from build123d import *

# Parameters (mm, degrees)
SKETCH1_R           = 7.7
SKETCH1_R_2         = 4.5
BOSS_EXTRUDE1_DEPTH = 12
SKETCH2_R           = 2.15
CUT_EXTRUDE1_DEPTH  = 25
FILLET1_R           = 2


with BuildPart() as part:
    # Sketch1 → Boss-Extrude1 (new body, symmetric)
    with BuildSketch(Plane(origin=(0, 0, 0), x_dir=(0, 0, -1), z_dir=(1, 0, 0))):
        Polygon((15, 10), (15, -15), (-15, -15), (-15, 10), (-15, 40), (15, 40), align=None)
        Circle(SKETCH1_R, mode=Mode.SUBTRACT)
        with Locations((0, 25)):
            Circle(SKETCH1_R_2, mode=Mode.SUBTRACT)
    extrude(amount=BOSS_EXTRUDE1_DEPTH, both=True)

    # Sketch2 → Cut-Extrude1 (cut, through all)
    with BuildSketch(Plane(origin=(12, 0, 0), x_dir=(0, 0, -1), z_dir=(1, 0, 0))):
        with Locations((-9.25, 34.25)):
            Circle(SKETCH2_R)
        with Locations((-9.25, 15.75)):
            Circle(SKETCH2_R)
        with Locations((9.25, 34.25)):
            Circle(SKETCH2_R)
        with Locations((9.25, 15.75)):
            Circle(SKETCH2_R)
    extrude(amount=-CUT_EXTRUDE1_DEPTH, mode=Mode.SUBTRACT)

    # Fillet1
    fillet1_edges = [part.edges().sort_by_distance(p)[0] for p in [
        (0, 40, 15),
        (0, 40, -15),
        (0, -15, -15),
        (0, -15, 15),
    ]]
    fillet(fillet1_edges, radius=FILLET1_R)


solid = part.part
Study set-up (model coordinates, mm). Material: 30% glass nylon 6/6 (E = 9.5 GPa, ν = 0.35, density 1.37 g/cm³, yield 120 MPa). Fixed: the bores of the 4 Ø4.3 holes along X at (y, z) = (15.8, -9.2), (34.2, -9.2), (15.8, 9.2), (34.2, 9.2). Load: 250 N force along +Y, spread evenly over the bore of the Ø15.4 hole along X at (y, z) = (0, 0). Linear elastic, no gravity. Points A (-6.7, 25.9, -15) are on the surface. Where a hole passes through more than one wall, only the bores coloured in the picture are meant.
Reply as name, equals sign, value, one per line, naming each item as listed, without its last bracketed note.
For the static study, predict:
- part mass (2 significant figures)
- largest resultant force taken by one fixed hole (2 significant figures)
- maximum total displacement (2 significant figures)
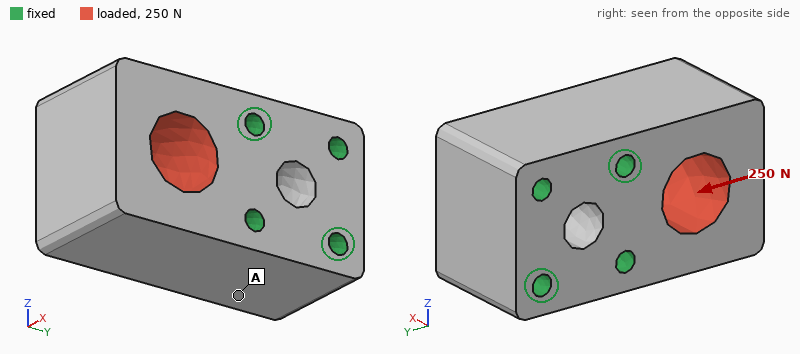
part mass = 44 g
largest resultant force taken by one fixed hole = 120 N
maximum total displacement = 1.8 µm
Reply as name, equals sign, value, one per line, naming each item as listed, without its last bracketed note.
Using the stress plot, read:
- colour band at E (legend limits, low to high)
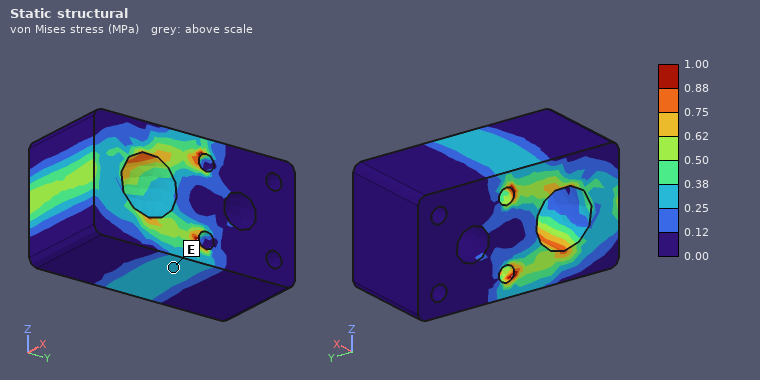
colour band at E = 0.25 to 0.38 MPa
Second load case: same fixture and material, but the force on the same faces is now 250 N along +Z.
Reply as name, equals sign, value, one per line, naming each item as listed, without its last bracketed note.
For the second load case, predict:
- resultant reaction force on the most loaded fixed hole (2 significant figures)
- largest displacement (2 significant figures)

resultant reaction force on the most loaded fixed hole = 190 N
largest displacement = 7.9 µm
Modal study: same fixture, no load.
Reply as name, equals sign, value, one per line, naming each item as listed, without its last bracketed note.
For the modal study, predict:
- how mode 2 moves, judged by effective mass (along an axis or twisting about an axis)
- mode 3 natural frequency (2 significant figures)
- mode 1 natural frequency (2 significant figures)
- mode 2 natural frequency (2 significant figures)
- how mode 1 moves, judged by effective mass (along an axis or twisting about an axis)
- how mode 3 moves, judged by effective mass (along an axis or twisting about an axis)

how mode 2 moves, judged by effective mass = along X
mode 3 natural frequency = 10 kHz
mode 1 natural frequency = 6500 Hz
mode 2 natural frequency = 7000 Hz
how mode 1 moves, judged by effective mass = along Z
how mode 3 moves, judged by effective mass = twisting about Y
